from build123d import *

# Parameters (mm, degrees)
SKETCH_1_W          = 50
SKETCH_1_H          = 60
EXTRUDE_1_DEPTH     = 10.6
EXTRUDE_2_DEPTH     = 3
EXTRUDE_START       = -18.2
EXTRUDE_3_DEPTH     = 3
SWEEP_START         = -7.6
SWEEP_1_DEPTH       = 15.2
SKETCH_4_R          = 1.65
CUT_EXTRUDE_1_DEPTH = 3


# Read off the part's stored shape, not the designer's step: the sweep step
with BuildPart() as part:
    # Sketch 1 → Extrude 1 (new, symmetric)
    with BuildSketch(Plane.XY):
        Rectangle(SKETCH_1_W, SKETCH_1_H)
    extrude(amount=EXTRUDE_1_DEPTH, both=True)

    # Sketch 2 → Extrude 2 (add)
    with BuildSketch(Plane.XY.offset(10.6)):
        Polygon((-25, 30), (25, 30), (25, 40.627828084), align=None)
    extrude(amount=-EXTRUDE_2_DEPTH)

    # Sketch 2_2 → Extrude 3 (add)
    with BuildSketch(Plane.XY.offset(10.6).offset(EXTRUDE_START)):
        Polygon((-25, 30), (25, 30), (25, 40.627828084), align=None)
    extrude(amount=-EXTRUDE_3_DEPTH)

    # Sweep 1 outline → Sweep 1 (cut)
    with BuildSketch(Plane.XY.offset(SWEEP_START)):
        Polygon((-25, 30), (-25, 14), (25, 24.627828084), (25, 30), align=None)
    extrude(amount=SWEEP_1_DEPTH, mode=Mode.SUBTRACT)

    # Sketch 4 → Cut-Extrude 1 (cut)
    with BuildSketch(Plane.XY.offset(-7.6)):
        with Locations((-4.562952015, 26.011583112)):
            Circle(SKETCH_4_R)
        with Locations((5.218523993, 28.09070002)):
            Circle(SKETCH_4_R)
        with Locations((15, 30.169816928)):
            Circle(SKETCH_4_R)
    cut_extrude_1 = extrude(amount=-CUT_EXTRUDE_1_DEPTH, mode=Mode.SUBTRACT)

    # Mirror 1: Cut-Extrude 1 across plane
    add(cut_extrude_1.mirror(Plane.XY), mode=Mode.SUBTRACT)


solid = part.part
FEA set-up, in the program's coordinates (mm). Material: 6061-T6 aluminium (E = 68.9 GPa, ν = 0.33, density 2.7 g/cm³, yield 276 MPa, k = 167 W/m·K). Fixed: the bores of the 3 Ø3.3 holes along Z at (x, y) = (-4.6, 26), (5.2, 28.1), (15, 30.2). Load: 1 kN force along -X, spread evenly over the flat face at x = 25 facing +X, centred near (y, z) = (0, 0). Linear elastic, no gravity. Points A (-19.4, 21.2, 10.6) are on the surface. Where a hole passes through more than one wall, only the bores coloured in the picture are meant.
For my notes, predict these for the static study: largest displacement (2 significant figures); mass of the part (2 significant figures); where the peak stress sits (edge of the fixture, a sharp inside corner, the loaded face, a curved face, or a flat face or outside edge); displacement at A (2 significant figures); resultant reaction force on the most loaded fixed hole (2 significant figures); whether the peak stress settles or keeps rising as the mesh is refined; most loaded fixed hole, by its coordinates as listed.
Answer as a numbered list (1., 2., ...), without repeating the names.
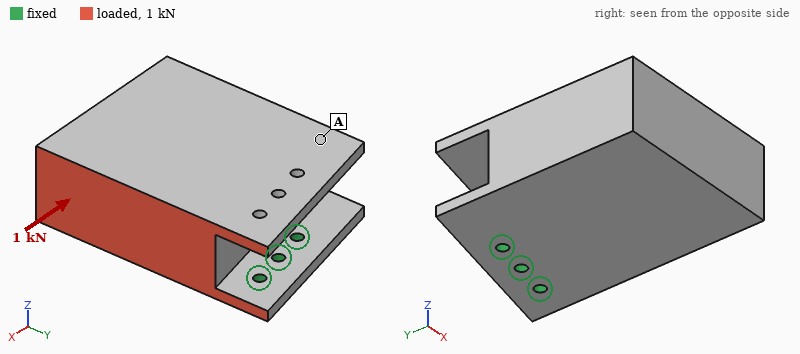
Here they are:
1. 0.14 mm
2. 150 g
3. edge of the fixture
4. 0.064 mm
5. 1.4 kN
6. keeps rising
7. (-4.6, 26)
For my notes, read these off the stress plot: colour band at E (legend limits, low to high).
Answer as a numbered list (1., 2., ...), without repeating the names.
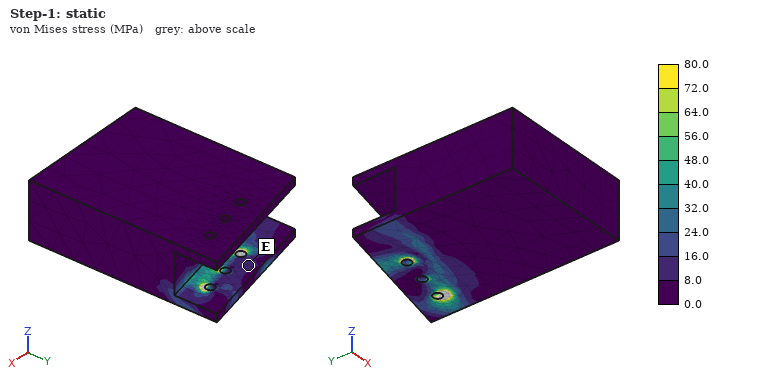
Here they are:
1. 8.0 to 16.0 MPa
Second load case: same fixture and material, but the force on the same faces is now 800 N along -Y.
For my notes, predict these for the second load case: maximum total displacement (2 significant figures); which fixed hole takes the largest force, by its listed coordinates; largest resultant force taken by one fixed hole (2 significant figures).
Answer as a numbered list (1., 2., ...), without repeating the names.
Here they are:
1. 0.52 mm
2. (15, 30.2)
3. 1.0 kN
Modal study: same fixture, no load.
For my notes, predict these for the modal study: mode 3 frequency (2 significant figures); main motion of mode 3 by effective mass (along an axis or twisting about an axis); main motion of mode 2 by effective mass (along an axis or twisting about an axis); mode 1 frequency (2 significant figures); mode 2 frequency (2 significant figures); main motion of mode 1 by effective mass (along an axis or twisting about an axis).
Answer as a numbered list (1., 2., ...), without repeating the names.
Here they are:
1. 2500 Hz
2. along X
3. along X
4. 360 Hz
5. 1800 Hz
6. along Z
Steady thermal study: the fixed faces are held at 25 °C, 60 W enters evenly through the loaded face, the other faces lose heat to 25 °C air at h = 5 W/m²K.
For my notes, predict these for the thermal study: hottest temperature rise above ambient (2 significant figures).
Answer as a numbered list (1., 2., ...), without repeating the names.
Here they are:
1. 41 K
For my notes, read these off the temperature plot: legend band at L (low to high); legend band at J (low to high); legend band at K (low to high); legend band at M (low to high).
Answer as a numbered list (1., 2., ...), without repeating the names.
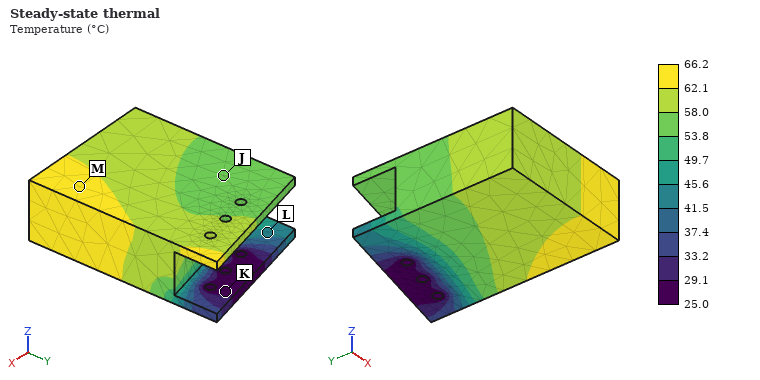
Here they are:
1. 41.5 to 45.6 °C
2. 53.8 to 58.0 °C
3. 25.0 to 29.1 °C
4. 62.1 to 66.2 °C
